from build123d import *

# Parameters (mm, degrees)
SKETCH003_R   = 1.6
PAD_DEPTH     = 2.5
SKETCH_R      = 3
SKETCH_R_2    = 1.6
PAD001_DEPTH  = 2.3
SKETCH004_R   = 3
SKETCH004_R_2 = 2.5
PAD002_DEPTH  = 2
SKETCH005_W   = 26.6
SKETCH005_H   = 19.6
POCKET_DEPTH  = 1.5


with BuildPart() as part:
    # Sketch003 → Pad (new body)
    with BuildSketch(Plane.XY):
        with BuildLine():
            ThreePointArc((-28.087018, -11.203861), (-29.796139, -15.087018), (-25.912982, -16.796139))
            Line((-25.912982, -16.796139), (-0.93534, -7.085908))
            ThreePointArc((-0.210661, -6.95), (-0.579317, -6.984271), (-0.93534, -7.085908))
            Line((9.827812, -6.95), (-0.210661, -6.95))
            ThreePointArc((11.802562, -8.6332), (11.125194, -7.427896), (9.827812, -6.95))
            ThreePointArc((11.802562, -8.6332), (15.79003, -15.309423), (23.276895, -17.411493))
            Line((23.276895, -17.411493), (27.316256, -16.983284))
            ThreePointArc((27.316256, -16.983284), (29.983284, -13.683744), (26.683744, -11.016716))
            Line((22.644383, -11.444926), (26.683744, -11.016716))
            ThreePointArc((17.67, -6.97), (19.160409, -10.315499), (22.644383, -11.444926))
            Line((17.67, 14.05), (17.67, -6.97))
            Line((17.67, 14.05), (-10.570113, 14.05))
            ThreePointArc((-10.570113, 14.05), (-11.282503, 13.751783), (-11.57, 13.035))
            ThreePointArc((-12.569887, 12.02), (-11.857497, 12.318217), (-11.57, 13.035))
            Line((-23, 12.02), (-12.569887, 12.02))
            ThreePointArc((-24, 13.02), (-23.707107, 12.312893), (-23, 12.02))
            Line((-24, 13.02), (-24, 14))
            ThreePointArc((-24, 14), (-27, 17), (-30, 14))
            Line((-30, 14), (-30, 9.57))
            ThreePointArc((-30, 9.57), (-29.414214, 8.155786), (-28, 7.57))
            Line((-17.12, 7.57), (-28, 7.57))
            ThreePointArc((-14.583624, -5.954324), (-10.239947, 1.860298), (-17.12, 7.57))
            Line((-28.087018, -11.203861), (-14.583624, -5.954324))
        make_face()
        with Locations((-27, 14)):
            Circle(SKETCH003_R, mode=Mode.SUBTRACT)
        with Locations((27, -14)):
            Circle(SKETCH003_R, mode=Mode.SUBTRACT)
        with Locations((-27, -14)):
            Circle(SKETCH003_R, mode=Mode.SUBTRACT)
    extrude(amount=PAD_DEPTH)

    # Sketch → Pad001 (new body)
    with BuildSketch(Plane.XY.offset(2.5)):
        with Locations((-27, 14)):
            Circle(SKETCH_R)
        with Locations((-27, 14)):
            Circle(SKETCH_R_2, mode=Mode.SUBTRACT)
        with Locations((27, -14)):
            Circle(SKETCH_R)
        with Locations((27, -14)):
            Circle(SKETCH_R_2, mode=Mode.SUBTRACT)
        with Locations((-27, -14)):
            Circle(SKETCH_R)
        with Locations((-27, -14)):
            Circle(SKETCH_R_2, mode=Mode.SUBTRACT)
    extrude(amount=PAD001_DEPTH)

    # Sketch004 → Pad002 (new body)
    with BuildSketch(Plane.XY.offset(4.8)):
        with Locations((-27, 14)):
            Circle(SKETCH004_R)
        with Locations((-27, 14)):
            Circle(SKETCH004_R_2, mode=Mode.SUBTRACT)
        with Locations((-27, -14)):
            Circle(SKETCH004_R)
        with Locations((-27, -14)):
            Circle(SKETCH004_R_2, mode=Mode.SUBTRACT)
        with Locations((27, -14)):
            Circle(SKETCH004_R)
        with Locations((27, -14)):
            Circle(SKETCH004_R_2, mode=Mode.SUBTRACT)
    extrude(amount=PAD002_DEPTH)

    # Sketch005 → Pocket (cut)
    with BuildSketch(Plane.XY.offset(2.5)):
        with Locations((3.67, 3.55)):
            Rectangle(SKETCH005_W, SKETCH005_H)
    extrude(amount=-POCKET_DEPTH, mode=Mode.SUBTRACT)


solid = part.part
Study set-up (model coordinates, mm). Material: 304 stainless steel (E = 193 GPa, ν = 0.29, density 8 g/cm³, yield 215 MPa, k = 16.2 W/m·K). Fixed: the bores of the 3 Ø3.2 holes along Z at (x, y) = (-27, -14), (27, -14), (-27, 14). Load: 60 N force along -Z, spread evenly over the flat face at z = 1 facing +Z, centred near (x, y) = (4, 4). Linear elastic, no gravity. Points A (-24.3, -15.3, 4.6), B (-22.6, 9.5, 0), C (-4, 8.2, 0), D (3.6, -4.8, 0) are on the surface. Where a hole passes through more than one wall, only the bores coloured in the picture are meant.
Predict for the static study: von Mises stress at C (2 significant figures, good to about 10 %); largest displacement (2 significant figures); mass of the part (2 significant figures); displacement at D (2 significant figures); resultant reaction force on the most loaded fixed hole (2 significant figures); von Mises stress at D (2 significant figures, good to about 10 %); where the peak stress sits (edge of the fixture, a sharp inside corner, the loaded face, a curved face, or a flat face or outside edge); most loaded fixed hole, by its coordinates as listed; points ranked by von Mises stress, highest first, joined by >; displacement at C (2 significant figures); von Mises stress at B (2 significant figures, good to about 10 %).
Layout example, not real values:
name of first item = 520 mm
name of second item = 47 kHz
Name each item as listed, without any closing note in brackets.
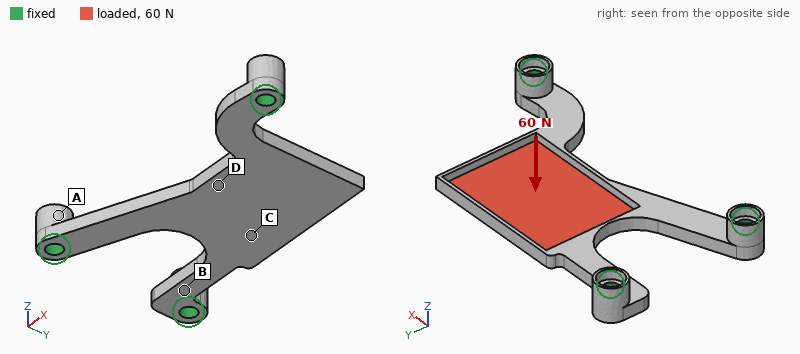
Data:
von Mises stress at C = 21 MPa
largest displacement = 0.11 mm
mass of the part = 14 g
displacement at D = 0.032 mm
resultant reaction force on the most loaded fixed hole = 88 N
von Mises stress at D = 29 MPa
where the peak stress sits = a curved face
most loaded fixed hole, by its coordinates as listed = (-27, 14)
points ranked by von Mises stress, highest first, joined by > = B > D > C > A
displacement at C = 0.047 mm
von Mises stress at B = 56 MPa
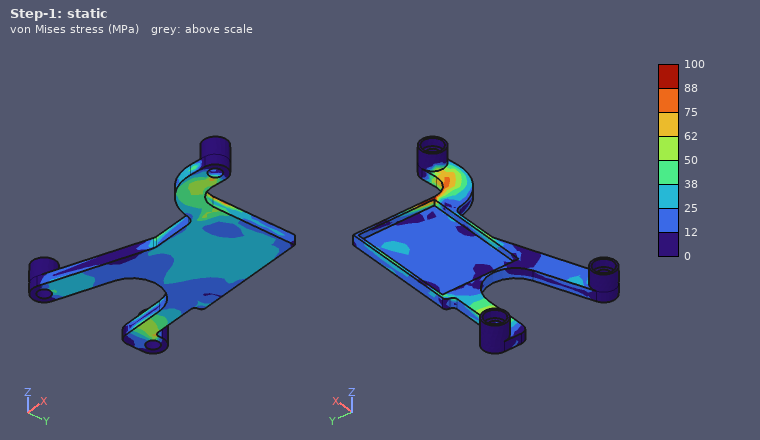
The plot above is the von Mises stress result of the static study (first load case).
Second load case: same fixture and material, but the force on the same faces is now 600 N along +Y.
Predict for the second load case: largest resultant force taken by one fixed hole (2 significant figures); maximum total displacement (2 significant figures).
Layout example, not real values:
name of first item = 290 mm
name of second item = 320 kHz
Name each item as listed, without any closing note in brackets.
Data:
largest resultant force taken by one fixed hole = 370 N
maximum total displacement = 19 µm
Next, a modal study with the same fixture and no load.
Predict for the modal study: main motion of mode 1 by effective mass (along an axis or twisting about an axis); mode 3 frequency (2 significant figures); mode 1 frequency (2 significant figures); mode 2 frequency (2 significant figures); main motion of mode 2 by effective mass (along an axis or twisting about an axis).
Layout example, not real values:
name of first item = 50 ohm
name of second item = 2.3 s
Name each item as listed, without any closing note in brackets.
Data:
main motion of mode 1 by effective mass = along Z
mode 3 frequency = 6100 Hz
mode 1 frequency = 2100 Hz
mode 2 frequency = 4900 Hz
main motion of mode 2 by effective mass = along Z
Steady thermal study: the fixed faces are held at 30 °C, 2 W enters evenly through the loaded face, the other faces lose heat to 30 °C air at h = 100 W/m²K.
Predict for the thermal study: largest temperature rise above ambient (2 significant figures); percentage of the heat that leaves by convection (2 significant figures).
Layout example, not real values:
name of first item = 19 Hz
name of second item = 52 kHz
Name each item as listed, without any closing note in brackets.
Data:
largest temperature rise above ambient = 19 K
percentage of the heat that leaves by convection = 87 %
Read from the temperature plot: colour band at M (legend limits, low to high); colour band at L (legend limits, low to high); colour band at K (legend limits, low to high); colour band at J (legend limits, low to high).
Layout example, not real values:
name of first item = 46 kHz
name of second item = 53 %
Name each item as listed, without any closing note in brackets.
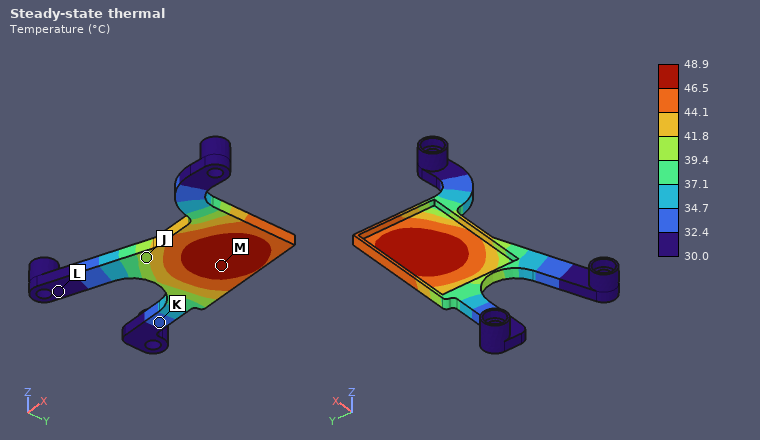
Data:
colour band at M = 46.5 to 48.9 °C
colour band at L = 30.0 to 32.4 °C
colour band at K = 32.4 to 34.7 °C
colour band at J = 39.4 to 41.8 °C
